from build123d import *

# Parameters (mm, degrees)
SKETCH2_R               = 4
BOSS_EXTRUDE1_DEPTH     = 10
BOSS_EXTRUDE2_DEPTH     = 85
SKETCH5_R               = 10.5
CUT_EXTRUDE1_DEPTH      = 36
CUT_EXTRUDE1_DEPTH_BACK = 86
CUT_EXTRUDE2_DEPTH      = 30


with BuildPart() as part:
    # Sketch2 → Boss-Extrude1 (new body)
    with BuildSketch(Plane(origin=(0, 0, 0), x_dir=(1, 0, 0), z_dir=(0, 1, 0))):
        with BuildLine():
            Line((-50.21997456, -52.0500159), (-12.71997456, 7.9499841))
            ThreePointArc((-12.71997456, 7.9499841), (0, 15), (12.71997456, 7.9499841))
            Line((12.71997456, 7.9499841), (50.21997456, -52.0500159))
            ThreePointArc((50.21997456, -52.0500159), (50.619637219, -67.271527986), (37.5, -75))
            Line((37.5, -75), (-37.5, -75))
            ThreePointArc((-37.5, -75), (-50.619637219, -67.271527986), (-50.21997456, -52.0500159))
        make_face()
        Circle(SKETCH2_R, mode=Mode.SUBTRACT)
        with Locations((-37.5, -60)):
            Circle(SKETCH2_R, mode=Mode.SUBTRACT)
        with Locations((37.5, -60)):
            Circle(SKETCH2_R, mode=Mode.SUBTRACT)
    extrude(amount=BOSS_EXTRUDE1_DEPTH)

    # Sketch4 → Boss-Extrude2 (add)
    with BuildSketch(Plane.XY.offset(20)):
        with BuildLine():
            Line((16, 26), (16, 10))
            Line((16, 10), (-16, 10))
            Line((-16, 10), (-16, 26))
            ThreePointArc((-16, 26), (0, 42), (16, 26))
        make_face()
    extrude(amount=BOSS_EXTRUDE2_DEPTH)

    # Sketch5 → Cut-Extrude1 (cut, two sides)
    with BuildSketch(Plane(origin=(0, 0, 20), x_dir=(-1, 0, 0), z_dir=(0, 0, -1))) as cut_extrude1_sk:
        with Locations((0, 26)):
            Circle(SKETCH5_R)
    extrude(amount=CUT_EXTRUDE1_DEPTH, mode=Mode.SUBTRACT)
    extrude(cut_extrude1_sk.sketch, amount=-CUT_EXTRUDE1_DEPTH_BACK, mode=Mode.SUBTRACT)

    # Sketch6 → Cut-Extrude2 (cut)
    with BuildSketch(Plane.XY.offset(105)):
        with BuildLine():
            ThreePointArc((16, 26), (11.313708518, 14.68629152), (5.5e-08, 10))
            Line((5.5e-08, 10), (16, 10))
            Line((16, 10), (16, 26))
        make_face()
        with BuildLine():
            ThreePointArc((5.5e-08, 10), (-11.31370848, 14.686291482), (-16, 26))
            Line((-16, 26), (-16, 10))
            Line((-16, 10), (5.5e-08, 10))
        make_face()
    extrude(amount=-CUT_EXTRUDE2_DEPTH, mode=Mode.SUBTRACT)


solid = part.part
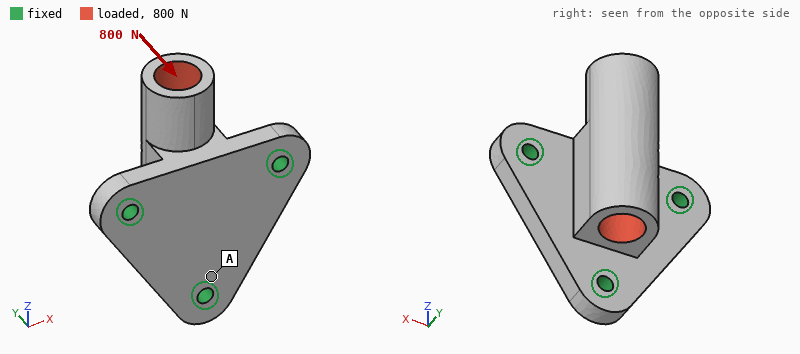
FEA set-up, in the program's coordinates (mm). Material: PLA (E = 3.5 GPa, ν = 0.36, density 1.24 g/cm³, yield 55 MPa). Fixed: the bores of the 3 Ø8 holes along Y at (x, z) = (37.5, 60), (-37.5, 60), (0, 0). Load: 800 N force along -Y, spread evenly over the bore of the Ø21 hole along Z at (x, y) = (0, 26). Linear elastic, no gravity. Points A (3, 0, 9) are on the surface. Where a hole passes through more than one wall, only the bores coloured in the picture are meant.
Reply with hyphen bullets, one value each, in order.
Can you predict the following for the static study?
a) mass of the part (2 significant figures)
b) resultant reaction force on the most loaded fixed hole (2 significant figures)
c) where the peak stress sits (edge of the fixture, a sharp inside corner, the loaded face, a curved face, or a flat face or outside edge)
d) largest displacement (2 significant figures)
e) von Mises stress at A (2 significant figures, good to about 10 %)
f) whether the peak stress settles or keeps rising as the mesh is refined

- 130 g
- 420 N
- edge of the fixture
- 0.25 mm
- 1.1 MPa
- keeps rising
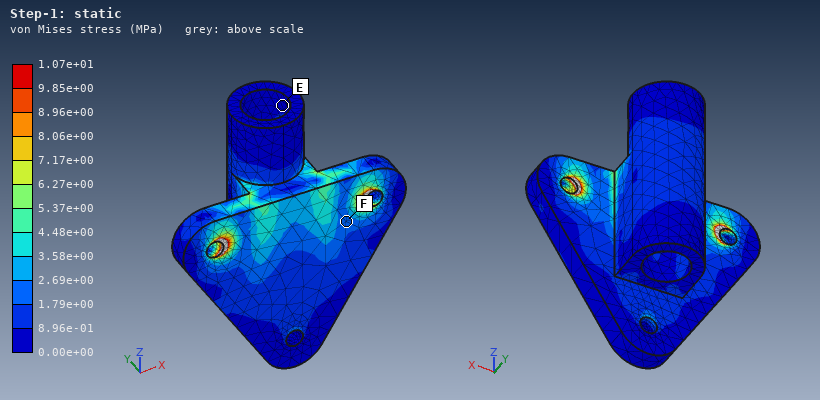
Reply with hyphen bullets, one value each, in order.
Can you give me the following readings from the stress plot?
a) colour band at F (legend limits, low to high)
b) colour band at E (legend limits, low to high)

- 1.79e+00 to 2.69e+00 MPa
- 0.00e+00 to 8.96e-01 MPa
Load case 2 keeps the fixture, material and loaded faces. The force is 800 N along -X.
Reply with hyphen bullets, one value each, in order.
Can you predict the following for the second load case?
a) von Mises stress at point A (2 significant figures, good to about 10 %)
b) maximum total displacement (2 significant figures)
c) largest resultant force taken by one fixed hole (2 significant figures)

- 1.1 MPa
- 0.17 mm
- 460 N
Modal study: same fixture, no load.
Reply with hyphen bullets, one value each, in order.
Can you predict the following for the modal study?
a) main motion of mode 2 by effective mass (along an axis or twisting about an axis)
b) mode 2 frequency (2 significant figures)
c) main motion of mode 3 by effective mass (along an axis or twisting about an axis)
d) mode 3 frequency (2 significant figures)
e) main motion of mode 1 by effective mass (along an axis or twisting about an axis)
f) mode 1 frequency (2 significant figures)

- along X
- 1900 Hz
- along Y
- 2300 Hz
- along Y
- 1400 Hz
